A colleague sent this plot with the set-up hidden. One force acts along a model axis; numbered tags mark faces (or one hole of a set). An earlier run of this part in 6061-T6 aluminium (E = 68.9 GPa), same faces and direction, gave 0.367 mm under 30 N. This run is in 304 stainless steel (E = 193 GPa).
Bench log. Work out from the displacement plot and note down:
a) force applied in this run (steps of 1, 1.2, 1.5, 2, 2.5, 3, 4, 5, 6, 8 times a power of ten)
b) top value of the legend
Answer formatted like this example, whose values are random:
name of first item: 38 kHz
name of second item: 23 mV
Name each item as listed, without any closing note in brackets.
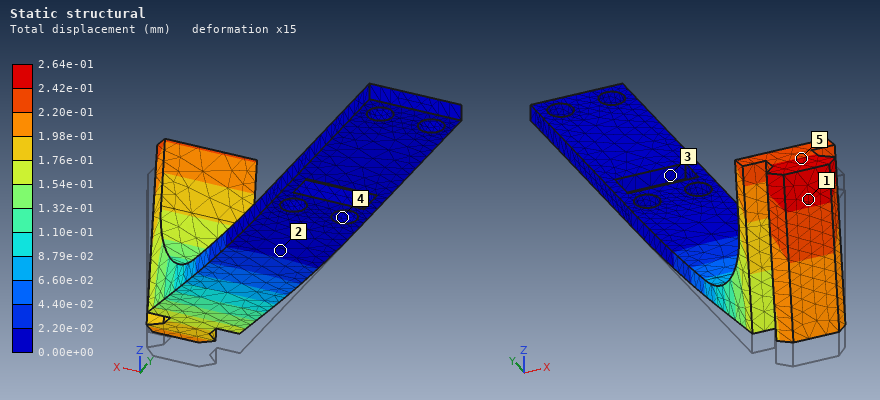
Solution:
force applied in this run: 60 N
top value of the legend: 2.64e-01 mm
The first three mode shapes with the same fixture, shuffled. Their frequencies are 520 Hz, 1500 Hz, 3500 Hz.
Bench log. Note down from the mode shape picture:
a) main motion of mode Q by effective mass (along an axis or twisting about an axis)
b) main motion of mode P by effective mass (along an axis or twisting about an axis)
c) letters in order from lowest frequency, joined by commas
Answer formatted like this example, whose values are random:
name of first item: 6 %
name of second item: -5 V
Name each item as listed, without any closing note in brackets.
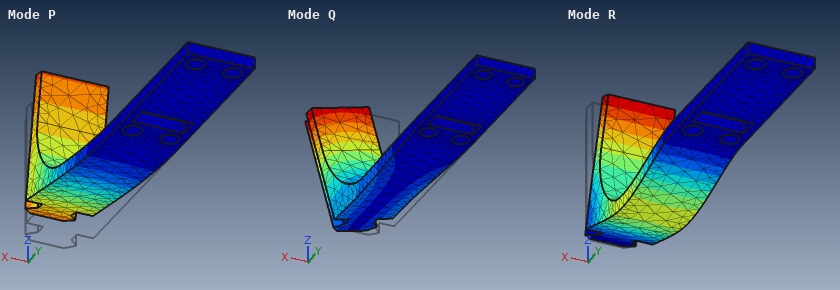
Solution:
main motion of mode Q by effective mass: along X
main motion of mode P by effective mass: along Z
letters in order from lowest frequency, joined by commas: P, Q, R
